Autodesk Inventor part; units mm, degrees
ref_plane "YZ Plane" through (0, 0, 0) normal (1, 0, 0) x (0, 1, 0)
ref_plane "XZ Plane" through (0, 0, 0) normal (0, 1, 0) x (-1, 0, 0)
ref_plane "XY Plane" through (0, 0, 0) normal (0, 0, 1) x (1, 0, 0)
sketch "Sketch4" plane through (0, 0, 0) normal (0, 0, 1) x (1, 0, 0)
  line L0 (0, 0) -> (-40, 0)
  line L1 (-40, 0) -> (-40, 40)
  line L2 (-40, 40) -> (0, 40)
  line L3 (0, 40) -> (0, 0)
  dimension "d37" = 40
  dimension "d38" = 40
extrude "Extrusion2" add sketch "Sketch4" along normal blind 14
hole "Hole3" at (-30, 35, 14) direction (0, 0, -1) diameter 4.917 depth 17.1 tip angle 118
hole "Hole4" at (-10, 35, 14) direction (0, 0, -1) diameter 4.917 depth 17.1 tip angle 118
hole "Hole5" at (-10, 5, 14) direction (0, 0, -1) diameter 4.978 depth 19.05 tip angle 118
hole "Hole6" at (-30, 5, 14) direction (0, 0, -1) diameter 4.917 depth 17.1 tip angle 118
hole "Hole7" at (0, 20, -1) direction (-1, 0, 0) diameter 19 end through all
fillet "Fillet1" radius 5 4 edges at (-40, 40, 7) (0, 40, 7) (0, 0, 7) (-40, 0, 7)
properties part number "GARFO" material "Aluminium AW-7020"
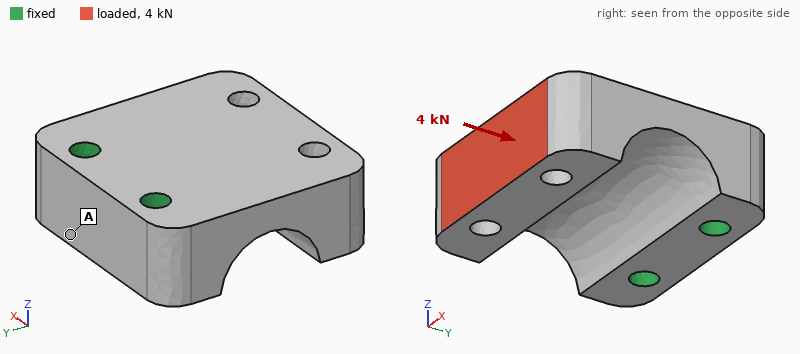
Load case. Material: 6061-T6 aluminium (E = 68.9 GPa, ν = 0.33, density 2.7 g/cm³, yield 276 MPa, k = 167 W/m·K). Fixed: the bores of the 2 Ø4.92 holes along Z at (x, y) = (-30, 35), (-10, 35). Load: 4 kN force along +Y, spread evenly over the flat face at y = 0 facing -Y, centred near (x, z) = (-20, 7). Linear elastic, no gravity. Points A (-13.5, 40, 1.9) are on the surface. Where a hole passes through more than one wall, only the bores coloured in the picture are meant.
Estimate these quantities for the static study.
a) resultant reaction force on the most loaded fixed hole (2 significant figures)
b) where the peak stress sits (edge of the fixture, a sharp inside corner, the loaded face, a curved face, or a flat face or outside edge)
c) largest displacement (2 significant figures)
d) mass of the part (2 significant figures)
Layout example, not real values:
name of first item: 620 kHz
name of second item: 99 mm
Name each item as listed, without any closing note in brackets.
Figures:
resultant reaction force on the most loaded fixed hole: 2.0 kN
where the peak stress sits: a curved face
largest displacement: 0.11 mm
mass of the part: 44 g
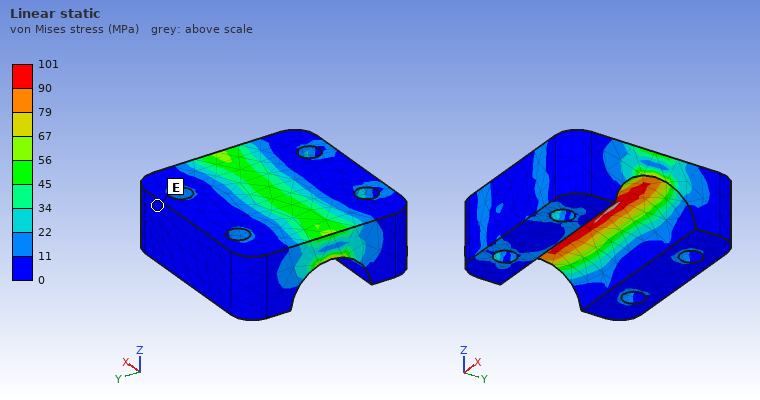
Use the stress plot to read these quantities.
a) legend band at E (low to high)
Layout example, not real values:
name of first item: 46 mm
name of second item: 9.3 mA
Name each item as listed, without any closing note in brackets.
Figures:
legend band at E: 0 to 11 MPa
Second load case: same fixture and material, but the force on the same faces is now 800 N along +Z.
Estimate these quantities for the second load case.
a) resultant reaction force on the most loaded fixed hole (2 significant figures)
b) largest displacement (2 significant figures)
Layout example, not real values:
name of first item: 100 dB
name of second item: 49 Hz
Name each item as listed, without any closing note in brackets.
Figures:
resultant reaction force on the most loaded fixed hole: 400 N
largest displacement: 0.13 mm
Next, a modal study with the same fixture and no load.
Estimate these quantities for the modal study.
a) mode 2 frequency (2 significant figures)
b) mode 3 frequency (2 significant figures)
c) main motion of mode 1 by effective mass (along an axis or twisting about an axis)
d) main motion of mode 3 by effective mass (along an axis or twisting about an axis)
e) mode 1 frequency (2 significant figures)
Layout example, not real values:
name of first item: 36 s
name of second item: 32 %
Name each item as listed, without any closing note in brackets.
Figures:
mode 2 frequency: 8900 Hz
mode 3 frequency: 12 kHz
main motion of mode 1 by effective mass: along Z
main motion of mode 3 by effective mass: along X
mode 1 frequency: 4100 Hz
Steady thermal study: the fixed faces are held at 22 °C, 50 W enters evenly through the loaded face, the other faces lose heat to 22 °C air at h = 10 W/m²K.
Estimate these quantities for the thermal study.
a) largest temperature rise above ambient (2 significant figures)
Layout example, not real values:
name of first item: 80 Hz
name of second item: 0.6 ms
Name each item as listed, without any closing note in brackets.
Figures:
largest temperature rise above ambient: 35 K
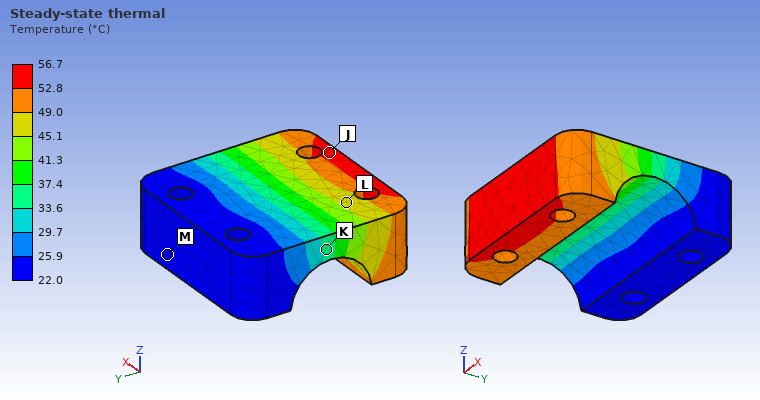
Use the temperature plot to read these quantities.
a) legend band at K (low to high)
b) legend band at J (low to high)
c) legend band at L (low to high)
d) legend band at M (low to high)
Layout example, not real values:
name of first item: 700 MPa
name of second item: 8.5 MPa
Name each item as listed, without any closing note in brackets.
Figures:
legend band at K: 33.6 to 37.4 °C
legend band at J: 52.8 to 56.7 °C
legend band at L: 45.1 to 49.0 °C
legend band at M: 22.0 to 25.9 °C
